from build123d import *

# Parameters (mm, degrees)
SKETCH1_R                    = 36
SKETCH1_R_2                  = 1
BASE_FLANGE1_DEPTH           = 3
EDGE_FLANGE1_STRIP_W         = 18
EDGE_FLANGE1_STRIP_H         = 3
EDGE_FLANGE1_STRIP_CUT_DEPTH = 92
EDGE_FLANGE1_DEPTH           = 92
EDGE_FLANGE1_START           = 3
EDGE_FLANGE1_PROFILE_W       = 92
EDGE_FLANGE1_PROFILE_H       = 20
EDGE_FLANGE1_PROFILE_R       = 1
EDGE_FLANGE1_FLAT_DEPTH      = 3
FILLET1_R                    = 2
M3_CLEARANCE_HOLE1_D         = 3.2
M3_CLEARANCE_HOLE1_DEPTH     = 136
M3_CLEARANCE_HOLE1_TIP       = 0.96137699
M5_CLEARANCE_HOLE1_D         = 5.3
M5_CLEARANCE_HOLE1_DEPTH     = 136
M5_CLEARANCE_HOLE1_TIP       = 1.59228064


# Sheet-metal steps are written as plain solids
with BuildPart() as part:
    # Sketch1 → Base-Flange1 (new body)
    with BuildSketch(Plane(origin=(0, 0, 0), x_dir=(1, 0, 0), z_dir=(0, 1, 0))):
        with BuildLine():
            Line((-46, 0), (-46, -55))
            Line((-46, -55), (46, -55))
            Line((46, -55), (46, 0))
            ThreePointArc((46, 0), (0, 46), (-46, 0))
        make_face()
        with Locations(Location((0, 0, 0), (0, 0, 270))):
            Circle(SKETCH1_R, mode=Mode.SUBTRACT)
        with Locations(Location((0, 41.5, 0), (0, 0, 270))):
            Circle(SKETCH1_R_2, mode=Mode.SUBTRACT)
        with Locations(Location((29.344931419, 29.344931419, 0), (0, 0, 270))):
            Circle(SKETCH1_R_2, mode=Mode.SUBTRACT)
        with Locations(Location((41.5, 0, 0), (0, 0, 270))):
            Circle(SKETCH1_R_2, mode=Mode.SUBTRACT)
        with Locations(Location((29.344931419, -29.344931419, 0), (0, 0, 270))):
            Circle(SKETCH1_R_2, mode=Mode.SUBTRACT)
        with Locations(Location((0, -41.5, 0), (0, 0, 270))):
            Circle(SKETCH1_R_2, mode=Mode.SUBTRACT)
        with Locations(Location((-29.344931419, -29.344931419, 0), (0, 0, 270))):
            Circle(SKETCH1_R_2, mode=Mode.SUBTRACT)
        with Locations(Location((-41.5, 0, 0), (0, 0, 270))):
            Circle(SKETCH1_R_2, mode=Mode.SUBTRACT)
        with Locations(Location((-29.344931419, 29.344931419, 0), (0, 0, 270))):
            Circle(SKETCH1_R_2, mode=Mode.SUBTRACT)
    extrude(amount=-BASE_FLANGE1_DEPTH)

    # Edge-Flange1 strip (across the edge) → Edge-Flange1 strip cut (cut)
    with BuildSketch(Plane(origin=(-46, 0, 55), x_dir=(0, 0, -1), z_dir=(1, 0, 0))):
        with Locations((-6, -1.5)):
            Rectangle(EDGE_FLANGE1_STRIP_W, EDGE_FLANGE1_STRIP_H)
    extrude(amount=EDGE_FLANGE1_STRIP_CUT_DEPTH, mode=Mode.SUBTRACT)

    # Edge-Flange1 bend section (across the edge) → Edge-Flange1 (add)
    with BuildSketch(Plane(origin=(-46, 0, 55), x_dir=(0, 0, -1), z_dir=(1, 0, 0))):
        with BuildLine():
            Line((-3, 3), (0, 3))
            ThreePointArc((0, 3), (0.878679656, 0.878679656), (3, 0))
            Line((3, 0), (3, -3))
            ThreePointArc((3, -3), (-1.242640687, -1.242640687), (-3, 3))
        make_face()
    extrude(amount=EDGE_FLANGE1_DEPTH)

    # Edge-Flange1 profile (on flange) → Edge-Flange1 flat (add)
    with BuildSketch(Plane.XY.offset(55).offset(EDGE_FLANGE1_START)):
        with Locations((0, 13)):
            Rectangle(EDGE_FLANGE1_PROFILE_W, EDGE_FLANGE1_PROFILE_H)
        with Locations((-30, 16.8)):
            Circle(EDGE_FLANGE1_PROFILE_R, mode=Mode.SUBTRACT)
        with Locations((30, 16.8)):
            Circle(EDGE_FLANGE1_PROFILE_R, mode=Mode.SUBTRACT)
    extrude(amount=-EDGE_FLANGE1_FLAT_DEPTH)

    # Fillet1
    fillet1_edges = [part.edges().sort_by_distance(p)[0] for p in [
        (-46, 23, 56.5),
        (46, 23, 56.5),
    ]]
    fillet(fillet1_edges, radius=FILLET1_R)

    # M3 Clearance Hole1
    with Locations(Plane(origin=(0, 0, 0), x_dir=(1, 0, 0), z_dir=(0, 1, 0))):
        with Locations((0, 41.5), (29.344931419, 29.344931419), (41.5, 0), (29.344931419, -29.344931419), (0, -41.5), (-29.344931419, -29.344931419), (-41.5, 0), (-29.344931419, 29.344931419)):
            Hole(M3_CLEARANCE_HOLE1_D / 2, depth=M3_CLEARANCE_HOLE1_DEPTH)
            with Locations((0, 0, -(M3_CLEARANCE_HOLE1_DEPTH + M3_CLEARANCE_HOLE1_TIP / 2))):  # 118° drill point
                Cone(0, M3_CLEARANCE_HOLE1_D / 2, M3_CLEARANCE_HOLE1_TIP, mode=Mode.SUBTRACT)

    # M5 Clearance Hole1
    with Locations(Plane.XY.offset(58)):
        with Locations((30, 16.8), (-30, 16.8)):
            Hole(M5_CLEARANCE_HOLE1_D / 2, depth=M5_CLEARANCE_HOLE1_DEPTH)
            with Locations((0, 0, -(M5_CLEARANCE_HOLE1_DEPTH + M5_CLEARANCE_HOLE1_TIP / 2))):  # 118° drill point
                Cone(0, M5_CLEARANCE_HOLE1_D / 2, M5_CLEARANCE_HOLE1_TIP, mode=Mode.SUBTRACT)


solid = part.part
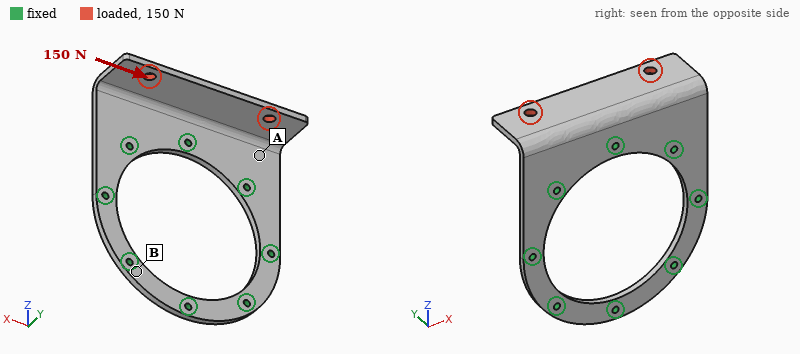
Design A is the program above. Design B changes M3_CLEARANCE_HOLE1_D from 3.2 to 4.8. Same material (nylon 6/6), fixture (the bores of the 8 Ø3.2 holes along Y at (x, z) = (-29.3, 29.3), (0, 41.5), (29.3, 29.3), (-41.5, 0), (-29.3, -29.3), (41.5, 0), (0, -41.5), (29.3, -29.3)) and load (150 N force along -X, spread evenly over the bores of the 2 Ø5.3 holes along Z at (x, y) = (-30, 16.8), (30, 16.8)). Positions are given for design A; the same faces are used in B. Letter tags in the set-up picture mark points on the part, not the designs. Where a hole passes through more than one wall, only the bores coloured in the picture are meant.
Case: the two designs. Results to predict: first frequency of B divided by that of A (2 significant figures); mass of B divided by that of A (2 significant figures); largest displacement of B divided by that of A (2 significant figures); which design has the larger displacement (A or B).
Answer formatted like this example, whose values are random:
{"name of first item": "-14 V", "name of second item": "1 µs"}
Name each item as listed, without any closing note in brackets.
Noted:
{"first frequency of B divided by that of A": "1.1", "mass of B divided by that of A": "0.99", "largest displacement of B divided by that of A": "0.90", "which design has the larger displacement": "A"}
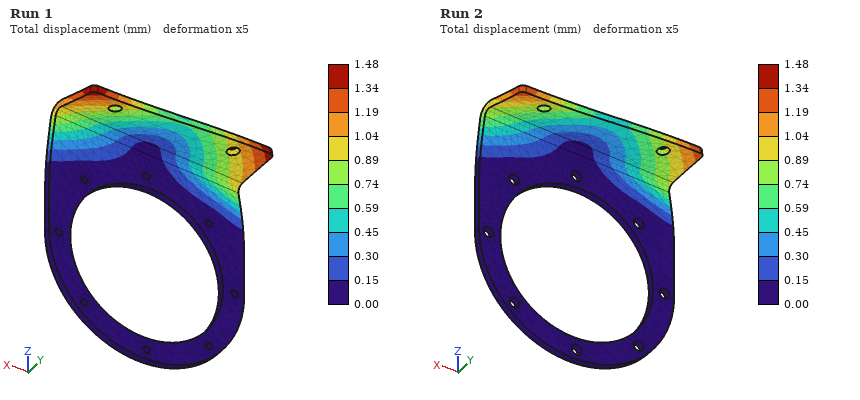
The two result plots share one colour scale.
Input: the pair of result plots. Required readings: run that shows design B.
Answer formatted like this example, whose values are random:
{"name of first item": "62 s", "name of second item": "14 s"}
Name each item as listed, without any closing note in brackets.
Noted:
{"run that shows design B": "Run 2"}
